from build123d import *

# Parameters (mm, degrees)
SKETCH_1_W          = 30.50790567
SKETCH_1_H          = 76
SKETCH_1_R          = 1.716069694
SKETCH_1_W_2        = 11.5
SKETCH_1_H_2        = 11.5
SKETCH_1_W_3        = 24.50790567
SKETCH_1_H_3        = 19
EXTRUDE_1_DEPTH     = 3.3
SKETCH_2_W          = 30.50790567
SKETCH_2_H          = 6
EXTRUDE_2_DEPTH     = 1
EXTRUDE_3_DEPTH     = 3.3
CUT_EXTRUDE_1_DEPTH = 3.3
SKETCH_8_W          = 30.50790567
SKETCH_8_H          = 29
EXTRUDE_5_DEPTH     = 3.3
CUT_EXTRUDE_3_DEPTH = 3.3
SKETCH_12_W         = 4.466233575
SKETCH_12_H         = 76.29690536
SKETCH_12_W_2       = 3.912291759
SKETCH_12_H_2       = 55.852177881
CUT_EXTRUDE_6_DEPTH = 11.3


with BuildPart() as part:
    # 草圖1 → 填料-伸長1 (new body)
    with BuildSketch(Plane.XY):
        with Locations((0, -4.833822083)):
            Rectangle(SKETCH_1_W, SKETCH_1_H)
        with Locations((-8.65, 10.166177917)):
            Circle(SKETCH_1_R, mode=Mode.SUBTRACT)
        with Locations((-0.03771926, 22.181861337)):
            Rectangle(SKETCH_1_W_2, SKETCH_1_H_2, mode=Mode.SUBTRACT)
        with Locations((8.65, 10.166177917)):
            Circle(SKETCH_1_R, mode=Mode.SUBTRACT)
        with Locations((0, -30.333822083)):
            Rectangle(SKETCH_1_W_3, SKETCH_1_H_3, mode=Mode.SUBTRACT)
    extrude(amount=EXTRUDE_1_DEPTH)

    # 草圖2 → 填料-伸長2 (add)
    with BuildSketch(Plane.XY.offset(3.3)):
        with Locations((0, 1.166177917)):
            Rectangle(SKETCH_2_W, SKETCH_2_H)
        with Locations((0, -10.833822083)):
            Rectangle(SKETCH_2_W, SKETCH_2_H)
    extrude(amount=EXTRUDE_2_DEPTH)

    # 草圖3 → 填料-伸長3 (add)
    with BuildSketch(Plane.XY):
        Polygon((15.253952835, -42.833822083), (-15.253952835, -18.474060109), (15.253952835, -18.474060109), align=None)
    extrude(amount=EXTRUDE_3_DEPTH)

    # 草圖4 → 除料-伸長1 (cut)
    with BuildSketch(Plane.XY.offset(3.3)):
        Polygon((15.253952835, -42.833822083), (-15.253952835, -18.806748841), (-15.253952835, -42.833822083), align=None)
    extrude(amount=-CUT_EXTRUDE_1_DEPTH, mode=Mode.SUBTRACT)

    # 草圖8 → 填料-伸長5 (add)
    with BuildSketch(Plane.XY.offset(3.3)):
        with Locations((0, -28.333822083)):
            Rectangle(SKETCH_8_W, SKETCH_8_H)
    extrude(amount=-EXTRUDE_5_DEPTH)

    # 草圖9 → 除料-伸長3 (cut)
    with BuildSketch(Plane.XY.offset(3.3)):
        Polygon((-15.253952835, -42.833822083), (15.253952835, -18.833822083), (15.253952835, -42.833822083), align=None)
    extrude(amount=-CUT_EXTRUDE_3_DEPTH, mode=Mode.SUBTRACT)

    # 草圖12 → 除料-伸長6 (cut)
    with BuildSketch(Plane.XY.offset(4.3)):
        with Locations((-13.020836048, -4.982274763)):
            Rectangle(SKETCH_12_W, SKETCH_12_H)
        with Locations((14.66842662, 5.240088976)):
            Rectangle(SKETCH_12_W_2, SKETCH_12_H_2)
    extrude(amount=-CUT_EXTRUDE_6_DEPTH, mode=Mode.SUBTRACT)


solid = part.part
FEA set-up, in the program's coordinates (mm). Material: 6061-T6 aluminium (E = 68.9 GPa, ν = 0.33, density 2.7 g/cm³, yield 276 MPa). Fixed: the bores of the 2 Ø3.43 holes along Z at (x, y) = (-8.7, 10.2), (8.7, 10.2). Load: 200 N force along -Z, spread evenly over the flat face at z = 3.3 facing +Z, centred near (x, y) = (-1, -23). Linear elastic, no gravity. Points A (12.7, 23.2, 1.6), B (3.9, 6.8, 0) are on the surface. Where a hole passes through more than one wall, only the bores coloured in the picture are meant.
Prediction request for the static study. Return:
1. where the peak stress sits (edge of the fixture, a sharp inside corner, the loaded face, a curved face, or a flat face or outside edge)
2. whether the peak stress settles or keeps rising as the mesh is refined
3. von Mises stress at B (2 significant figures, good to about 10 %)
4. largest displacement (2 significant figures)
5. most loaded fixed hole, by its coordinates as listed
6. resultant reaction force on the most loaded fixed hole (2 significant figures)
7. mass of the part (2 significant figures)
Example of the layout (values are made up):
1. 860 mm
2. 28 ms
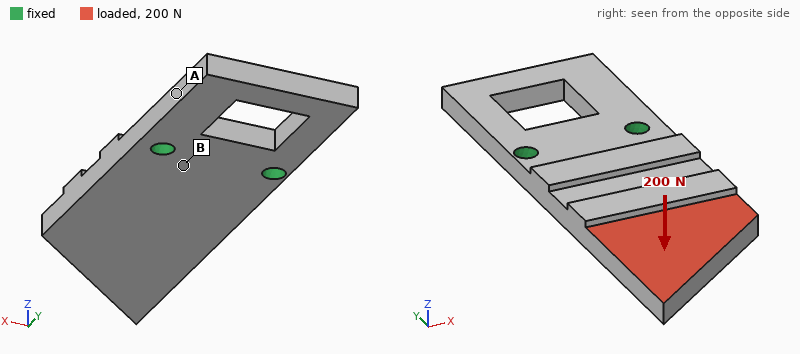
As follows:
1. edge of the fixture
2. keeps rising
3. 100 MPa
4. 0.74 mm
5. (-8.7, 10.2)
6. 110 N
7. 13 g
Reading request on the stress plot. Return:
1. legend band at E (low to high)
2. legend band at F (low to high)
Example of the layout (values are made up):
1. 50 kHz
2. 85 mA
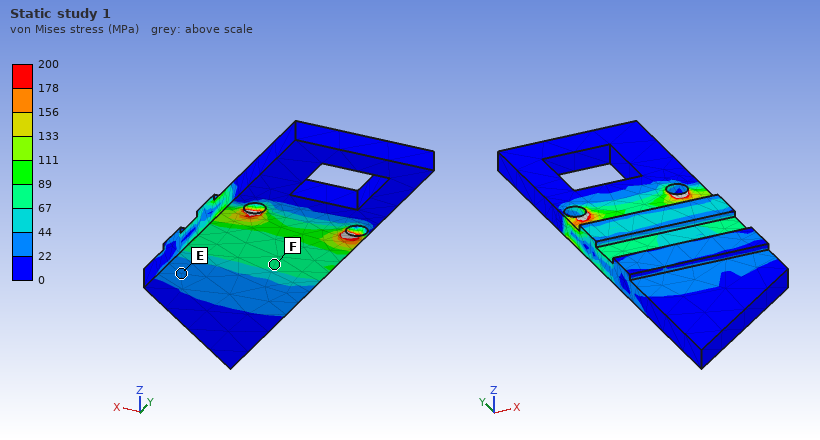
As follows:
1. 22 to 44 MPa
2. 67 to 89 MPa
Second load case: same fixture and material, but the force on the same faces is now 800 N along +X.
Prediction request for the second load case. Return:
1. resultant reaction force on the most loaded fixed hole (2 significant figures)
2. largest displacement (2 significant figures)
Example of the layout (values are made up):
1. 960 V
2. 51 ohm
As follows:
1. 1.5 kN
2. 0.10 mm
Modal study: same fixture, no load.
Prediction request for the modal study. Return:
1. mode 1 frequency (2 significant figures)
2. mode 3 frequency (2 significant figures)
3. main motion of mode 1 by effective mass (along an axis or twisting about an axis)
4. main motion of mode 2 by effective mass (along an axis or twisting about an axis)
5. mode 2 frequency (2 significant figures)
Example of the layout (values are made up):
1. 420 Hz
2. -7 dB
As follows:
1. 1700 Hz
2. 6700 Hz
3. along Z
4. along Z
5. 4600 Hz
